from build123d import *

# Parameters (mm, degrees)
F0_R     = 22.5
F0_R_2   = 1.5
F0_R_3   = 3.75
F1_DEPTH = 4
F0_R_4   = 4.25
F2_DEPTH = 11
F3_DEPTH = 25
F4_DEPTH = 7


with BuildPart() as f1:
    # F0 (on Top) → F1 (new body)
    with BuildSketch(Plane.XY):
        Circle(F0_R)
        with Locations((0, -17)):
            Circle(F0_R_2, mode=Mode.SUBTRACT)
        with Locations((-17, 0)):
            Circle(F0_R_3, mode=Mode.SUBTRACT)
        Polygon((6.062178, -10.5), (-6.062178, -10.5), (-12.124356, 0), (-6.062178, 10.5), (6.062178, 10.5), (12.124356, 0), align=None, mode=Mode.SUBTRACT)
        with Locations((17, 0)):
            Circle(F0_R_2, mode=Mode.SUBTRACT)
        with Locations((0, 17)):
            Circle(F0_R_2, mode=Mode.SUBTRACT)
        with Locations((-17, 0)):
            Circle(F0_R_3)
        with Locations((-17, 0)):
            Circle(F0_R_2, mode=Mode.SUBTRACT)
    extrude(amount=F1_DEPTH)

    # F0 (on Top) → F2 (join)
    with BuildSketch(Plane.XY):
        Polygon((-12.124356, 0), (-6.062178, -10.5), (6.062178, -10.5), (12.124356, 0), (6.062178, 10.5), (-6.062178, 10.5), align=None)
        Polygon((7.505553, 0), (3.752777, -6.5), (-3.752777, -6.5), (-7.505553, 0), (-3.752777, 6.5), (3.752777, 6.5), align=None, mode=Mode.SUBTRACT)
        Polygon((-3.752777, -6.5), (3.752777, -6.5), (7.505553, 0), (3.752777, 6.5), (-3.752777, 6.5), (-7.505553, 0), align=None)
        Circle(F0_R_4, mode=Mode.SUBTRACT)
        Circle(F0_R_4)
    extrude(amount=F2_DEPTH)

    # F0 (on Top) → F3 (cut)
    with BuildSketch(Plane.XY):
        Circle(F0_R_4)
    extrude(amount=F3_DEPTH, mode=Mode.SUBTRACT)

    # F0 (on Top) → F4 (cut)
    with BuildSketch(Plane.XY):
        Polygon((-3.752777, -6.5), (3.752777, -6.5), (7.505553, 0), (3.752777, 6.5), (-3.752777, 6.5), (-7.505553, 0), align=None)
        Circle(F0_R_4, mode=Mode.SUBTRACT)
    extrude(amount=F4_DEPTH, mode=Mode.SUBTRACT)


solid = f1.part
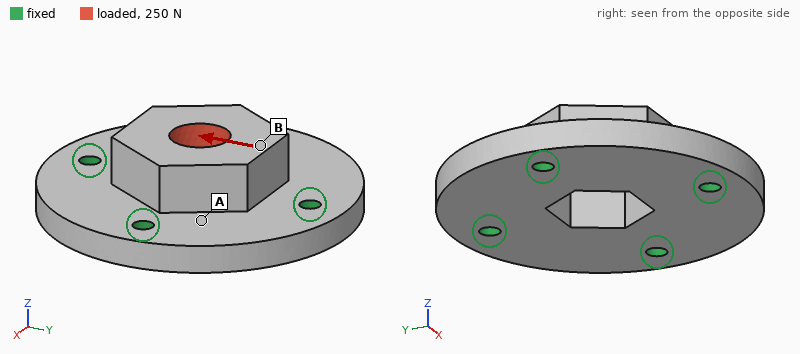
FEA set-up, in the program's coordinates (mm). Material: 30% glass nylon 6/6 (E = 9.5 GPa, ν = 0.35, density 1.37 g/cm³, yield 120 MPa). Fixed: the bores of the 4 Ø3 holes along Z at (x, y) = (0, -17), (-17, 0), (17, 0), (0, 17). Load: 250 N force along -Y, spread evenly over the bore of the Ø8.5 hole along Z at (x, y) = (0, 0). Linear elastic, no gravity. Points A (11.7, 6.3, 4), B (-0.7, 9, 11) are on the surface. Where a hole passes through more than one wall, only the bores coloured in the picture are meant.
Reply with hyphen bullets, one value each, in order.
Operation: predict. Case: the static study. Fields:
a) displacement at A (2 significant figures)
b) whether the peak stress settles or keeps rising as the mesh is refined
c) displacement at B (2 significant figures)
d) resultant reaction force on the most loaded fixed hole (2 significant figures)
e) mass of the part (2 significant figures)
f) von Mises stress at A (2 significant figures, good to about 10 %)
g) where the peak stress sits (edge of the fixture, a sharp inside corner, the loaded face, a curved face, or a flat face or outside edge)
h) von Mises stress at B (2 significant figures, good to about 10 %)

- 2.5 µm
- keeps rising
- 9.2 µm
- 94 N
- 11 g
- 1.0 MPa
- edge of the fixture
- 2.2 MPa
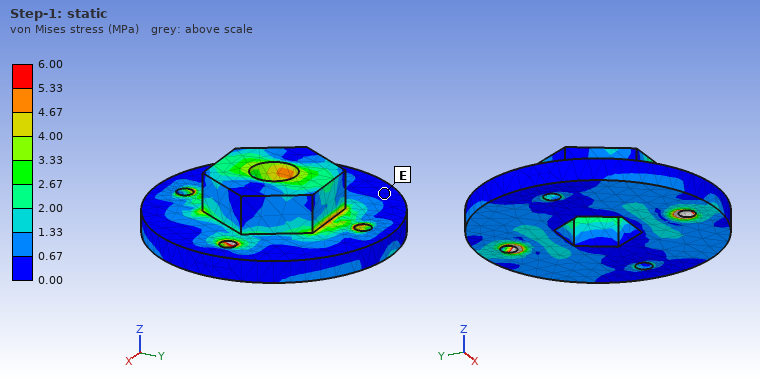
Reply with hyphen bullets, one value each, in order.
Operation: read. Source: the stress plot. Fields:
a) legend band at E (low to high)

- 0.00 to 0.67 MPa
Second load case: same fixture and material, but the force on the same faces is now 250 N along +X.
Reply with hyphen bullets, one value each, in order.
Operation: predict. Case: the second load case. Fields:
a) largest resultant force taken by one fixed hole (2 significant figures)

- 94 N
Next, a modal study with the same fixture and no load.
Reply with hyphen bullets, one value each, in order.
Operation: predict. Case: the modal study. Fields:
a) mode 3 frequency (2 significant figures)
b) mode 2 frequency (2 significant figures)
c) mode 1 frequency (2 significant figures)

- 12 kHz
- 12 kHz
- 12 kHz
